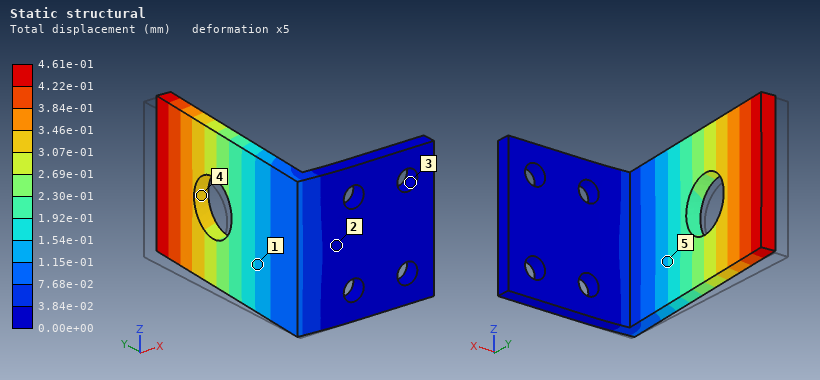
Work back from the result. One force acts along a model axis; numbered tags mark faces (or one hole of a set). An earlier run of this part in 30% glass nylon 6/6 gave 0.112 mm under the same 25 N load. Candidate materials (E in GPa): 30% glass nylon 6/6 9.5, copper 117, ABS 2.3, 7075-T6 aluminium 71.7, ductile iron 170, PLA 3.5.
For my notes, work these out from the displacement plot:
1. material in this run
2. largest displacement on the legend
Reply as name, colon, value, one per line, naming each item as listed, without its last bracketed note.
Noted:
material in this run: ABS
largest displacement on the legend: 4.61e-01 mm
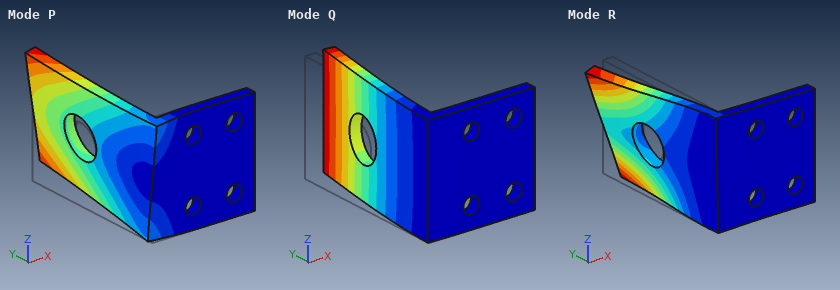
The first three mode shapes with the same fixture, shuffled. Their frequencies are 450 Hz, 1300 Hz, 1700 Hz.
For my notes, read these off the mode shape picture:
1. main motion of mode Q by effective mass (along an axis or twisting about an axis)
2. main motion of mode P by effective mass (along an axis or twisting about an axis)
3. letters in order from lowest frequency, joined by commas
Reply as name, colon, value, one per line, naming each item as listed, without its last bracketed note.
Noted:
main motion of mode Q by effective mass: along X
main motion of mode P by effective mass: along Z
letters in order from lowest frequency, joined by commas: Q, P, R
